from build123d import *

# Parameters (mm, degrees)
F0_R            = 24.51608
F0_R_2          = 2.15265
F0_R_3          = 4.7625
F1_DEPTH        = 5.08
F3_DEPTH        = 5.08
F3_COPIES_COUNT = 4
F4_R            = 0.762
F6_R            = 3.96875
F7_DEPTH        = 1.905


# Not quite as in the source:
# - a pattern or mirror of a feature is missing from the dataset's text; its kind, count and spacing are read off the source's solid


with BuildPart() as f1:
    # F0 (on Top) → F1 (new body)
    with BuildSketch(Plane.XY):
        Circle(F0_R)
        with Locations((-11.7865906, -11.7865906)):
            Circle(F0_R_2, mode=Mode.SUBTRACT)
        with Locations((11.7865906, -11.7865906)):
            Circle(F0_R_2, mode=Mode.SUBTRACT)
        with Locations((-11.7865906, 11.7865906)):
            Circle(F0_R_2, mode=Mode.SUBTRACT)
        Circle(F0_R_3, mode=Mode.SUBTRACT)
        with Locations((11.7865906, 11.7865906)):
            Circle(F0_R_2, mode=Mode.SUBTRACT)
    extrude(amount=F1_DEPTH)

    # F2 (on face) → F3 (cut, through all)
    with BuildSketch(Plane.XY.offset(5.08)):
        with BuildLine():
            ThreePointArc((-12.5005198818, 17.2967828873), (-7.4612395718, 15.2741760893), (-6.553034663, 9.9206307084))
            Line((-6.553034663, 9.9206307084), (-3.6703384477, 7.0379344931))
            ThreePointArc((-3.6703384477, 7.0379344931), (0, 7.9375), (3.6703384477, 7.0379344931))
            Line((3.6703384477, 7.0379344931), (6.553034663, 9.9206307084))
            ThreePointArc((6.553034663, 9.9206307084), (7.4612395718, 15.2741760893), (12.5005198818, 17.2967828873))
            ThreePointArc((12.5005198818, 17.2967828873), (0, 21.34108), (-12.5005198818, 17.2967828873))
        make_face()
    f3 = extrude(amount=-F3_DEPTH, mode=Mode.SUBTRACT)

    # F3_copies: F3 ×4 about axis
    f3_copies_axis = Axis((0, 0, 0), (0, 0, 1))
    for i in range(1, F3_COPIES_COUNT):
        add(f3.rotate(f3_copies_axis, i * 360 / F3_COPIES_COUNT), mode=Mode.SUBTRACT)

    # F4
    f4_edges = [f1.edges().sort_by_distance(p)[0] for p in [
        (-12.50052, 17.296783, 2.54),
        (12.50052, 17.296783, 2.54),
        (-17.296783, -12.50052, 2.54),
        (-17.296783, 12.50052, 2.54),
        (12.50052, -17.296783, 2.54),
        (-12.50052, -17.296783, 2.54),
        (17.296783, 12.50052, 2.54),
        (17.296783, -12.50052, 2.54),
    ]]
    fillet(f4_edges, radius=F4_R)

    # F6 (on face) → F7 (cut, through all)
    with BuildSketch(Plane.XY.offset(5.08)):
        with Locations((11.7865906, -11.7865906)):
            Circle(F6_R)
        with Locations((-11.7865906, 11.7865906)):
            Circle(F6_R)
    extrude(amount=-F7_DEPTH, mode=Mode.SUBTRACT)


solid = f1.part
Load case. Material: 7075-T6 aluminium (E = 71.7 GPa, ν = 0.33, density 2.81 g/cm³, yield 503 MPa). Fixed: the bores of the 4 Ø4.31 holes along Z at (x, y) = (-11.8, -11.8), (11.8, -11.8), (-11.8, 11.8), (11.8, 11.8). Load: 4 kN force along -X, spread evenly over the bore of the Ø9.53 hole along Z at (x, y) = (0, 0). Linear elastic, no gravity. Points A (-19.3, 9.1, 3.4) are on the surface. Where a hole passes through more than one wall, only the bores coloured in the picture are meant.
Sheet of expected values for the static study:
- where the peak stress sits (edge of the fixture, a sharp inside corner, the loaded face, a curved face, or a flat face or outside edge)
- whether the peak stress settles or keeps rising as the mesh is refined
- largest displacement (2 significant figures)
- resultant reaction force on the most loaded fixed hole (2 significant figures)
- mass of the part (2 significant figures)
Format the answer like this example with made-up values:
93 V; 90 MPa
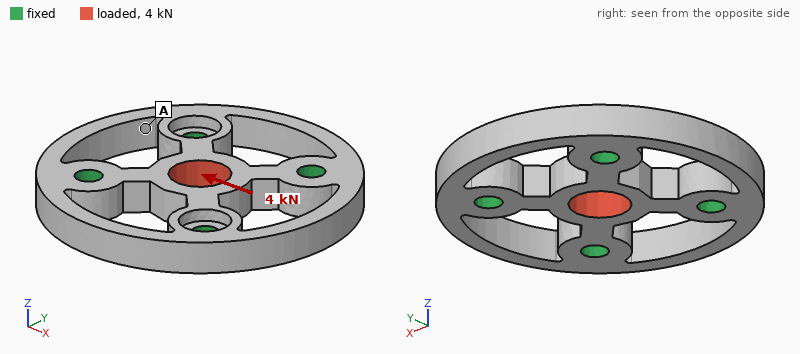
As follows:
edge of the fixture; keeps rising; 18 µm; 1.2 kN; 13 g
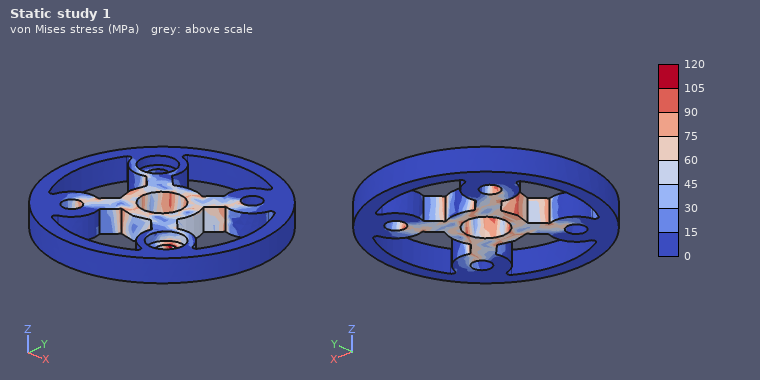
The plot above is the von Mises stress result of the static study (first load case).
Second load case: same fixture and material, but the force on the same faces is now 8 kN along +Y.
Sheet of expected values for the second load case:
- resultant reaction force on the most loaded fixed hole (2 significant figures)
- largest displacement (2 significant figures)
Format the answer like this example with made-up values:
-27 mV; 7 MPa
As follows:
2.4 kN; 35 µm
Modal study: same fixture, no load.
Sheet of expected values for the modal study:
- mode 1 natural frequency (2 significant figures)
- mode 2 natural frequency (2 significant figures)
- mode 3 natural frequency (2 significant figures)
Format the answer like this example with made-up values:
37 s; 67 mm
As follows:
16 kHz; 17 kHz; 18 kHz
